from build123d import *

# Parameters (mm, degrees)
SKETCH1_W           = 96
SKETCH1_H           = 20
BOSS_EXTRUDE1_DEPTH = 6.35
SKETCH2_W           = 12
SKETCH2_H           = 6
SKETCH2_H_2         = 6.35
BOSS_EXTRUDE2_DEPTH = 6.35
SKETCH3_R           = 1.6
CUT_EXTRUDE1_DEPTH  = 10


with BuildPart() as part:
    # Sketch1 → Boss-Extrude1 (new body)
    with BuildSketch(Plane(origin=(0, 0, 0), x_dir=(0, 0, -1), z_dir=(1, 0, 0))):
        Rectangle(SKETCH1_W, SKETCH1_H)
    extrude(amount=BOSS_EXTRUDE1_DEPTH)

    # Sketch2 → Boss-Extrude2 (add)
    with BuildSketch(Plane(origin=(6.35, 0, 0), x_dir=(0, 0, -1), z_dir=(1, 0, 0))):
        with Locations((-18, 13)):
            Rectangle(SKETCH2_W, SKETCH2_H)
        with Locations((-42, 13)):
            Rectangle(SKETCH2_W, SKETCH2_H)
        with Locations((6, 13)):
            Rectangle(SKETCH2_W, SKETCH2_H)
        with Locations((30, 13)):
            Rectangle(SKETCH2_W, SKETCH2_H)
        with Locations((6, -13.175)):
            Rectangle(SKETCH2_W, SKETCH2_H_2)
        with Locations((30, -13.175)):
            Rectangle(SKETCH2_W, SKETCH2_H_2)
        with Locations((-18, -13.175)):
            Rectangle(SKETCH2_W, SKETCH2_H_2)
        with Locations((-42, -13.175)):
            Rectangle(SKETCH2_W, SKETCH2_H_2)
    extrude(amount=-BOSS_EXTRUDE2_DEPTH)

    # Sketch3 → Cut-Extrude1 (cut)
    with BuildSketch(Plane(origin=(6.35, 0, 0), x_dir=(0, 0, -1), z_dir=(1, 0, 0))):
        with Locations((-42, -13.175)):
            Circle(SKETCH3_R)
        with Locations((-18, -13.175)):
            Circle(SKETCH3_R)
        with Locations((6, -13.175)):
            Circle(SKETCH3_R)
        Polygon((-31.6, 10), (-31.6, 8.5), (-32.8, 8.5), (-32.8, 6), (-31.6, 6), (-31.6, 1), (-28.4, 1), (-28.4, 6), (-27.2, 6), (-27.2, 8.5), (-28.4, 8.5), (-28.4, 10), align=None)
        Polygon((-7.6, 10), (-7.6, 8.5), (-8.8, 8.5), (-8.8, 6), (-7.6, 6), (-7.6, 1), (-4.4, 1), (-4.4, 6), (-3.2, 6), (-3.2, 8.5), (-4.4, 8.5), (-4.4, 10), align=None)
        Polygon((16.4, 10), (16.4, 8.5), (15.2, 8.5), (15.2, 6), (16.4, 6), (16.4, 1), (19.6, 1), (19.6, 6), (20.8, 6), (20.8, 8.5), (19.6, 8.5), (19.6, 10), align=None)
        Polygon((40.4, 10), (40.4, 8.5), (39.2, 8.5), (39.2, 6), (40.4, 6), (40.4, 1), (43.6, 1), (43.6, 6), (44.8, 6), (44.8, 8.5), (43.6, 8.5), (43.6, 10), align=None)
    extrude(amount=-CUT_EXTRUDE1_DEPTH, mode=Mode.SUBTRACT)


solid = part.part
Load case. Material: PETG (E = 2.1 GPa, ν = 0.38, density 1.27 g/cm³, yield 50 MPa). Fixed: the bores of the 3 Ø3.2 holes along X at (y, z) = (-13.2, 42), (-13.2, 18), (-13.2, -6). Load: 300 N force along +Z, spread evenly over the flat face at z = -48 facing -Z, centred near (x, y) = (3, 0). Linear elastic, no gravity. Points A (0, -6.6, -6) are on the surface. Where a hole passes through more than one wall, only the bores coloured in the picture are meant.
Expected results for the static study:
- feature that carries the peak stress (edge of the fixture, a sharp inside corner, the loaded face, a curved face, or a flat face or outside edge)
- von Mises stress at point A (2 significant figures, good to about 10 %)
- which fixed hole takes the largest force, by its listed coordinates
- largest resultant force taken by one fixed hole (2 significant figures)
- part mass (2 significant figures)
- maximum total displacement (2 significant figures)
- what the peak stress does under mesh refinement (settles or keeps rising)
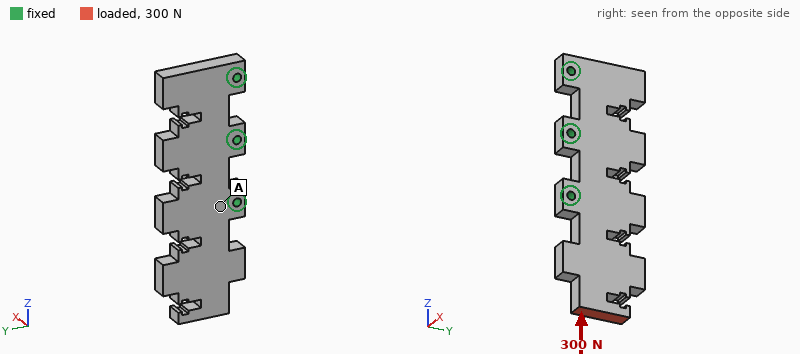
a sharp inside corner
3.3 MPa
(-13.2, 18)
170 N
19 g
1.0 mm
keeps rising
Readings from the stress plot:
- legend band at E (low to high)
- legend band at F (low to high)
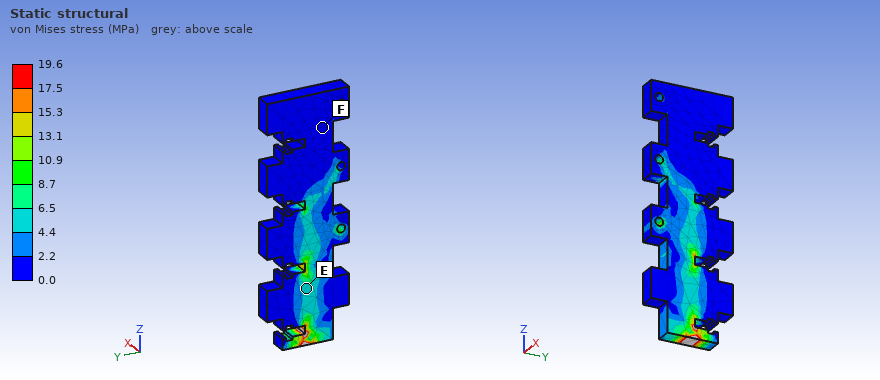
4.4 to 6.5 MPa
0.0 to 2.2 MPa
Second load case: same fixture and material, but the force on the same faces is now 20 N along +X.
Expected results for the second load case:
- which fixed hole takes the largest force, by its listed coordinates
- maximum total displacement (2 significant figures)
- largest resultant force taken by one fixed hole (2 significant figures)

(-13.2, -6)
1.1 mm
38 N
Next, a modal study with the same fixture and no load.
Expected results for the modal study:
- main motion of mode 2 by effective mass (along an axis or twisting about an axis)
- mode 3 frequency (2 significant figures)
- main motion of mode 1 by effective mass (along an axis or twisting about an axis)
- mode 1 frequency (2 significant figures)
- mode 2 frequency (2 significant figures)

along Y
1100 Hz
along X
510 Hz
980 Hz
